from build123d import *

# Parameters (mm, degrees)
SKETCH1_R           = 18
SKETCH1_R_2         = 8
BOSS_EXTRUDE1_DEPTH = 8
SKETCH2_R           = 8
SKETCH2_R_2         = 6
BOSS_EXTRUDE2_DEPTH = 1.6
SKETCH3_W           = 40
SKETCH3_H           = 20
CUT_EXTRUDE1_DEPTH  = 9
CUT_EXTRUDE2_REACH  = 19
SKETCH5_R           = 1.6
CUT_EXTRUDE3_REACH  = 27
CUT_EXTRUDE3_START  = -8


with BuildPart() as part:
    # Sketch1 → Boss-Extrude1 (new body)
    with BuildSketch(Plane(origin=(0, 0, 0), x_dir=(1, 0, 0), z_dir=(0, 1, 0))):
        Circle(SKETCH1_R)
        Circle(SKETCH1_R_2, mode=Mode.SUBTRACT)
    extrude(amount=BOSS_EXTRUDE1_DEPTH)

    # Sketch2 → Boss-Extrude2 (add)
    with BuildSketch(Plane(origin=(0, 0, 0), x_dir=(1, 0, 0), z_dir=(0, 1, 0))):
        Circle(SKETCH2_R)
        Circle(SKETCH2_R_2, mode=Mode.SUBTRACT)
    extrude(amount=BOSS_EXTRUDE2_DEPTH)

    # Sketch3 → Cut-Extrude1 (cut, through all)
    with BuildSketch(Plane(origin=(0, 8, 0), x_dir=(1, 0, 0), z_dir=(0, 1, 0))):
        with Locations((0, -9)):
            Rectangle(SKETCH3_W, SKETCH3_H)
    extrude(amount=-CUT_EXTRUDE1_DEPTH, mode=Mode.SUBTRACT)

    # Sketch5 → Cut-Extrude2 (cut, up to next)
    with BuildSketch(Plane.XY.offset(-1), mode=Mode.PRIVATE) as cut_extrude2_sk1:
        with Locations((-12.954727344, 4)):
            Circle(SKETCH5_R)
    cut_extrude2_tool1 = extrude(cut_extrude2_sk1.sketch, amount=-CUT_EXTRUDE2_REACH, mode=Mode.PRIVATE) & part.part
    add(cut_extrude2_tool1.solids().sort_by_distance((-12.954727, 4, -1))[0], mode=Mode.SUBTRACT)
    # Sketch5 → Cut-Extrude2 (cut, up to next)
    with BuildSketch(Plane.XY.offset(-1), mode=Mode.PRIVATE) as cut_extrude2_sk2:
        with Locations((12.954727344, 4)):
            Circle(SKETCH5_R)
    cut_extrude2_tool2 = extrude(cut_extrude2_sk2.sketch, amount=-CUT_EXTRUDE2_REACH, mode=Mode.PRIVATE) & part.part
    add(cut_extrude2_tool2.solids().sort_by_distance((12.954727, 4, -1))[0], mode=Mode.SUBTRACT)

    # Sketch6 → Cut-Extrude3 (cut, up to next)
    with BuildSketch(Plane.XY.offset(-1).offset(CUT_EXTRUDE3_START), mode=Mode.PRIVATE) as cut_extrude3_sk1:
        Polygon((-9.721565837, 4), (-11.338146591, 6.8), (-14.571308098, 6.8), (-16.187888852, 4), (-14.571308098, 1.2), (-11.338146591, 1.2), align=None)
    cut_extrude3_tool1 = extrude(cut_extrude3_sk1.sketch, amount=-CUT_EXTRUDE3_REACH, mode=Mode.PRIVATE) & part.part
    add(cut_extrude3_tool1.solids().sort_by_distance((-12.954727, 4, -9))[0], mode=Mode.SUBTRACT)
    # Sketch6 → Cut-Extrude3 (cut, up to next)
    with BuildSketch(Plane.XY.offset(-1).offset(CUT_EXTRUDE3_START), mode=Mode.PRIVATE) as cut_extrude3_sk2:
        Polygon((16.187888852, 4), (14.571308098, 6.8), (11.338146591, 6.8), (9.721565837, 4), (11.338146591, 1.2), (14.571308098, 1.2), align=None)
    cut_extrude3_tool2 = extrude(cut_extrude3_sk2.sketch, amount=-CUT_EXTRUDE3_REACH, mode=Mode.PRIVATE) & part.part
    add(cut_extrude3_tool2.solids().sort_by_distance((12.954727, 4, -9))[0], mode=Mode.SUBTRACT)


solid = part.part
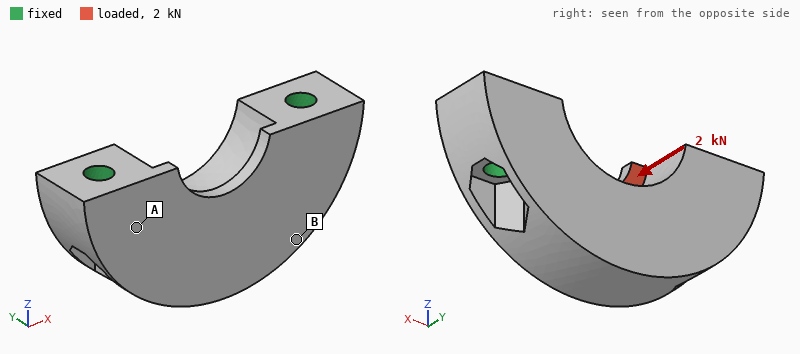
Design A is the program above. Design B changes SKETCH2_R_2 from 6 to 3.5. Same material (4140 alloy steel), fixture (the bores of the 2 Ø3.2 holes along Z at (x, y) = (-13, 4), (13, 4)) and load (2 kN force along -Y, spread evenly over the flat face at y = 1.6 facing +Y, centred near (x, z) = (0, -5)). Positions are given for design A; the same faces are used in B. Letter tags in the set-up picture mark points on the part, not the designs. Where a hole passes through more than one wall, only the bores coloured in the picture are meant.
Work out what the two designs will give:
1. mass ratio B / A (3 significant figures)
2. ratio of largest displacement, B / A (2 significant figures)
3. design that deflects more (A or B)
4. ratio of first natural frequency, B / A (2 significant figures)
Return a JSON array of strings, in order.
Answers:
["1.02", "2.8", "B", "1.0"]
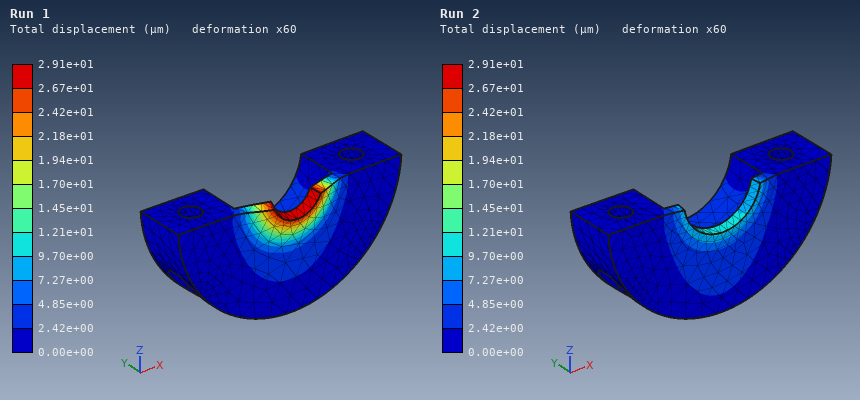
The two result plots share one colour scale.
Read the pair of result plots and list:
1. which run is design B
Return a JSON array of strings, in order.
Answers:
["Run 1"]
